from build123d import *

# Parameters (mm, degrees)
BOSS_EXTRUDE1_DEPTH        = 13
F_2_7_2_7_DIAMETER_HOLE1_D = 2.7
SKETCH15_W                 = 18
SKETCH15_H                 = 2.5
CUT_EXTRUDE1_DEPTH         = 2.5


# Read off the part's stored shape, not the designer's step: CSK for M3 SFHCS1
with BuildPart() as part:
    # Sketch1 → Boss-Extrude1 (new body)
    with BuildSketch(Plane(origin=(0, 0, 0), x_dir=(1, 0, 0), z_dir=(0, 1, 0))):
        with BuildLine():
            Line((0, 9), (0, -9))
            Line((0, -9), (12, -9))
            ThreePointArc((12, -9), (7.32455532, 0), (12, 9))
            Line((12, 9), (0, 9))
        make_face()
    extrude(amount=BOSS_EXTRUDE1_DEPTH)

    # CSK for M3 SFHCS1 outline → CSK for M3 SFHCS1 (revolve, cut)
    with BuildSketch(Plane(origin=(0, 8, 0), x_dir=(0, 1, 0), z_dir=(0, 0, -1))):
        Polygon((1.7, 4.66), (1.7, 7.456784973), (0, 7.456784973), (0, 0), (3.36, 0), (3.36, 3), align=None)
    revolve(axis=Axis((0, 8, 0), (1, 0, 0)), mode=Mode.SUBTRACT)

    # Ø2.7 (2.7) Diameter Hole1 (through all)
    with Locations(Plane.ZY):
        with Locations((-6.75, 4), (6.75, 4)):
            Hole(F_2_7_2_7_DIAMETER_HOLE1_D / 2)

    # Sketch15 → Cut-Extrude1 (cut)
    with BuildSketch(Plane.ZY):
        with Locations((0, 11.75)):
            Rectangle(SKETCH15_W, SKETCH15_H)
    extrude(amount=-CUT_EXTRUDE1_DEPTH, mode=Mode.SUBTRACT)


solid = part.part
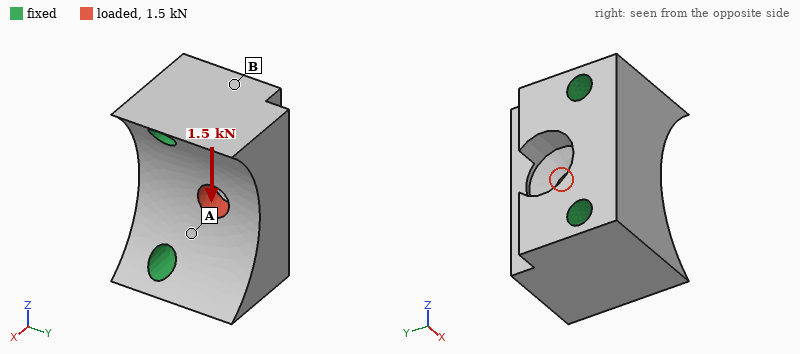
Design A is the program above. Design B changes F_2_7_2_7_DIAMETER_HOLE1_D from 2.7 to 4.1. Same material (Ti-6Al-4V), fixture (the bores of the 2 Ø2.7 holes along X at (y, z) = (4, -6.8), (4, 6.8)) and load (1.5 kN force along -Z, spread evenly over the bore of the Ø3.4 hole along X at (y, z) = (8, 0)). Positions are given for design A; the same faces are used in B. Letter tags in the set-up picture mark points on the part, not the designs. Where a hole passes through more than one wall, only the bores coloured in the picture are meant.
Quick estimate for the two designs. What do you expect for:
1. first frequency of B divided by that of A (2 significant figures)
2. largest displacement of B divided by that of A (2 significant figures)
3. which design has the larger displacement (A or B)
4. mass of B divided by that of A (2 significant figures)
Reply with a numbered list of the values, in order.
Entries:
1. 1.1
2. 0.87
3. A
4. 0.91
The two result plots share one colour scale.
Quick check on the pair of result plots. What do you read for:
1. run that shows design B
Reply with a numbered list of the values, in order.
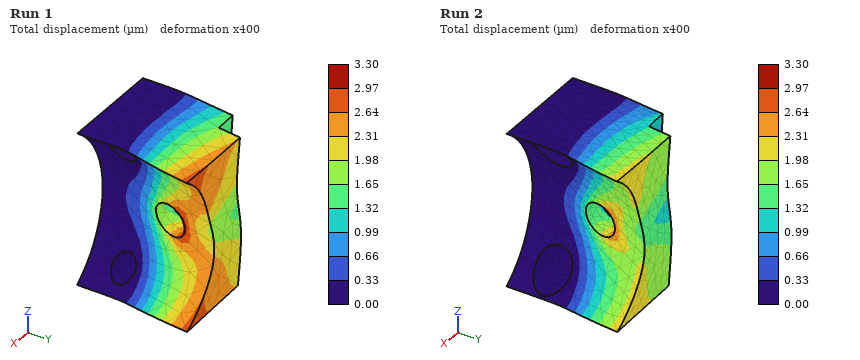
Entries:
1. Run 2
